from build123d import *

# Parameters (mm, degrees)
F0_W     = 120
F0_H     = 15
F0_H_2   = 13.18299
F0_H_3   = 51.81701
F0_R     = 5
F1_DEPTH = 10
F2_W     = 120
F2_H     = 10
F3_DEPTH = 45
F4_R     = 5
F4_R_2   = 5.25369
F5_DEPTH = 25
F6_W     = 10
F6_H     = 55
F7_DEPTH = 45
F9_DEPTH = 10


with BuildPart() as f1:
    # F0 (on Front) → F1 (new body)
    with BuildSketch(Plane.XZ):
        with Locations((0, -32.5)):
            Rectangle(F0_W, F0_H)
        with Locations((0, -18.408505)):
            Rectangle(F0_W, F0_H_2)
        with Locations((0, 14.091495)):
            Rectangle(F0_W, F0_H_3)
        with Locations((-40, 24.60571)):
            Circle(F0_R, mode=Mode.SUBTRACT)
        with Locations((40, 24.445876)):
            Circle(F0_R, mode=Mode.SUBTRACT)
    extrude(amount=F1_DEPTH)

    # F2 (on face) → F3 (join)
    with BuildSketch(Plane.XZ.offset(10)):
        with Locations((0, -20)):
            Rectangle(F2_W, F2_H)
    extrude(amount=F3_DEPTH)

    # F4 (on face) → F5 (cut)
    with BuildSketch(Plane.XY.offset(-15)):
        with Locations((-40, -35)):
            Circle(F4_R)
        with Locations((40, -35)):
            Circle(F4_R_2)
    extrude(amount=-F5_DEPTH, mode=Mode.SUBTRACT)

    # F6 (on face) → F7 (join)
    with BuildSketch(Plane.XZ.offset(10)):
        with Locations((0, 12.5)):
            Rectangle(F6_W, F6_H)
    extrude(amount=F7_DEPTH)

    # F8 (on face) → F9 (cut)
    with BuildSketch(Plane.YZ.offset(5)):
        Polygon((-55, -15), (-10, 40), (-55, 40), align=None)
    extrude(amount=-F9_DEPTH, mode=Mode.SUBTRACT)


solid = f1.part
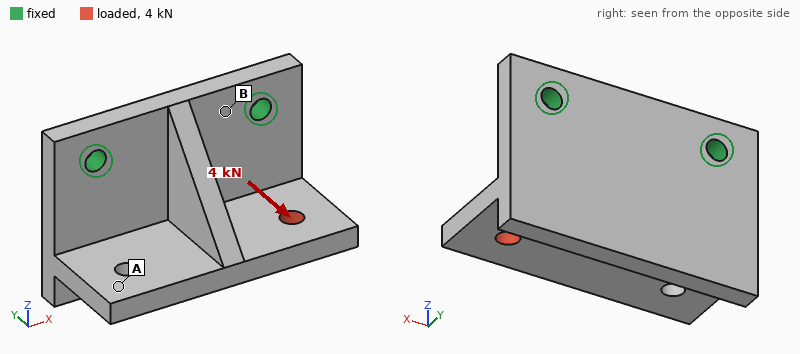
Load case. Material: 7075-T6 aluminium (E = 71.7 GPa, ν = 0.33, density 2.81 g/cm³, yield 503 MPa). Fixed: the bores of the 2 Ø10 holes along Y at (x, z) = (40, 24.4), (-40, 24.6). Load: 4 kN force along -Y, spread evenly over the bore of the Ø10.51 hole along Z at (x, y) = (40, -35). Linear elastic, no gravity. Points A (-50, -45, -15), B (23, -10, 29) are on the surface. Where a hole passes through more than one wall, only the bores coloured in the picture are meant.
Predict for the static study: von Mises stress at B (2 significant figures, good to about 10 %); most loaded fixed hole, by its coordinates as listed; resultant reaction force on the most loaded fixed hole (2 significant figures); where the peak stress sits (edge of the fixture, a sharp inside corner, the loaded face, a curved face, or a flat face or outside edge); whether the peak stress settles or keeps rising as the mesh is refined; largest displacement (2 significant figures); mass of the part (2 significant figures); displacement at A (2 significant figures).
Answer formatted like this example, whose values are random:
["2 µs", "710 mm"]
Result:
["44 MPa", "(40, 24.4)", "3.9 kN", "edge of the fixture", "keeps rising", "0.40 mm", "450 g", "0.17 mm"]
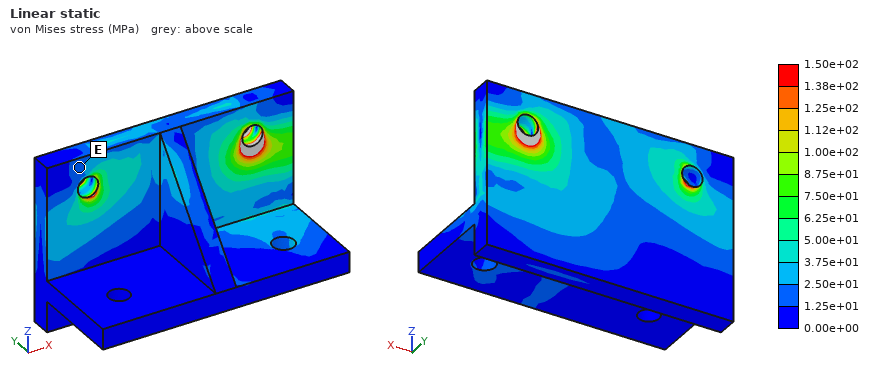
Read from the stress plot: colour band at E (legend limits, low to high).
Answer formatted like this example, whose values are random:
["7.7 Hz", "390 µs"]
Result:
["1.25e+01 to 2.50e+01 MPa"]
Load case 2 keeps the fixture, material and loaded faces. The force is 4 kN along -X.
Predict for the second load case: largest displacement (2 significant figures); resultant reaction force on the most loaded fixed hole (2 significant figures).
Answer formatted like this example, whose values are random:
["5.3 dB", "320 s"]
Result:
["0.10 mm", "3.2 kN"]
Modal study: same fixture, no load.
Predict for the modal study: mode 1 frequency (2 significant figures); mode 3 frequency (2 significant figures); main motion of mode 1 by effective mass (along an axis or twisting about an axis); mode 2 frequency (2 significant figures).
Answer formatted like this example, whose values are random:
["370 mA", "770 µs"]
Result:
["1200 Hz", "4200 Hz", "along Y", "2200 Hz"]
